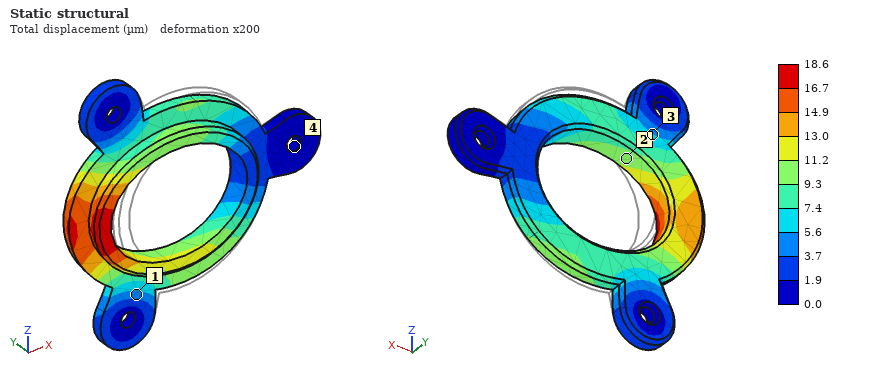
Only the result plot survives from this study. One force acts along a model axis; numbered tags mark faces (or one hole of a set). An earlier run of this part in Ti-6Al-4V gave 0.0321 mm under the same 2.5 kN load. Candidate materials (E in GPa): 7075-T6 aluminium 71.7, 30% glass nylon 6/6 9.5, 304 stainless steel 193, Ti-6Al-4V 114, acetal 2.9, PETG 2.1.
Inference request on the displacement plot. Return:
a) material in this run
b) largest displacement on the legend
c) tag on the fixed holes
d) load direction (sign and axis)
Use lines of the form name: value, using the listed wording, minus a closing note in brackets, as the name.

material in this run: 304 stainless steel
largest displacement on the legend: 18.6 µm
tag on the fixed holes: 4
load direction: -X
